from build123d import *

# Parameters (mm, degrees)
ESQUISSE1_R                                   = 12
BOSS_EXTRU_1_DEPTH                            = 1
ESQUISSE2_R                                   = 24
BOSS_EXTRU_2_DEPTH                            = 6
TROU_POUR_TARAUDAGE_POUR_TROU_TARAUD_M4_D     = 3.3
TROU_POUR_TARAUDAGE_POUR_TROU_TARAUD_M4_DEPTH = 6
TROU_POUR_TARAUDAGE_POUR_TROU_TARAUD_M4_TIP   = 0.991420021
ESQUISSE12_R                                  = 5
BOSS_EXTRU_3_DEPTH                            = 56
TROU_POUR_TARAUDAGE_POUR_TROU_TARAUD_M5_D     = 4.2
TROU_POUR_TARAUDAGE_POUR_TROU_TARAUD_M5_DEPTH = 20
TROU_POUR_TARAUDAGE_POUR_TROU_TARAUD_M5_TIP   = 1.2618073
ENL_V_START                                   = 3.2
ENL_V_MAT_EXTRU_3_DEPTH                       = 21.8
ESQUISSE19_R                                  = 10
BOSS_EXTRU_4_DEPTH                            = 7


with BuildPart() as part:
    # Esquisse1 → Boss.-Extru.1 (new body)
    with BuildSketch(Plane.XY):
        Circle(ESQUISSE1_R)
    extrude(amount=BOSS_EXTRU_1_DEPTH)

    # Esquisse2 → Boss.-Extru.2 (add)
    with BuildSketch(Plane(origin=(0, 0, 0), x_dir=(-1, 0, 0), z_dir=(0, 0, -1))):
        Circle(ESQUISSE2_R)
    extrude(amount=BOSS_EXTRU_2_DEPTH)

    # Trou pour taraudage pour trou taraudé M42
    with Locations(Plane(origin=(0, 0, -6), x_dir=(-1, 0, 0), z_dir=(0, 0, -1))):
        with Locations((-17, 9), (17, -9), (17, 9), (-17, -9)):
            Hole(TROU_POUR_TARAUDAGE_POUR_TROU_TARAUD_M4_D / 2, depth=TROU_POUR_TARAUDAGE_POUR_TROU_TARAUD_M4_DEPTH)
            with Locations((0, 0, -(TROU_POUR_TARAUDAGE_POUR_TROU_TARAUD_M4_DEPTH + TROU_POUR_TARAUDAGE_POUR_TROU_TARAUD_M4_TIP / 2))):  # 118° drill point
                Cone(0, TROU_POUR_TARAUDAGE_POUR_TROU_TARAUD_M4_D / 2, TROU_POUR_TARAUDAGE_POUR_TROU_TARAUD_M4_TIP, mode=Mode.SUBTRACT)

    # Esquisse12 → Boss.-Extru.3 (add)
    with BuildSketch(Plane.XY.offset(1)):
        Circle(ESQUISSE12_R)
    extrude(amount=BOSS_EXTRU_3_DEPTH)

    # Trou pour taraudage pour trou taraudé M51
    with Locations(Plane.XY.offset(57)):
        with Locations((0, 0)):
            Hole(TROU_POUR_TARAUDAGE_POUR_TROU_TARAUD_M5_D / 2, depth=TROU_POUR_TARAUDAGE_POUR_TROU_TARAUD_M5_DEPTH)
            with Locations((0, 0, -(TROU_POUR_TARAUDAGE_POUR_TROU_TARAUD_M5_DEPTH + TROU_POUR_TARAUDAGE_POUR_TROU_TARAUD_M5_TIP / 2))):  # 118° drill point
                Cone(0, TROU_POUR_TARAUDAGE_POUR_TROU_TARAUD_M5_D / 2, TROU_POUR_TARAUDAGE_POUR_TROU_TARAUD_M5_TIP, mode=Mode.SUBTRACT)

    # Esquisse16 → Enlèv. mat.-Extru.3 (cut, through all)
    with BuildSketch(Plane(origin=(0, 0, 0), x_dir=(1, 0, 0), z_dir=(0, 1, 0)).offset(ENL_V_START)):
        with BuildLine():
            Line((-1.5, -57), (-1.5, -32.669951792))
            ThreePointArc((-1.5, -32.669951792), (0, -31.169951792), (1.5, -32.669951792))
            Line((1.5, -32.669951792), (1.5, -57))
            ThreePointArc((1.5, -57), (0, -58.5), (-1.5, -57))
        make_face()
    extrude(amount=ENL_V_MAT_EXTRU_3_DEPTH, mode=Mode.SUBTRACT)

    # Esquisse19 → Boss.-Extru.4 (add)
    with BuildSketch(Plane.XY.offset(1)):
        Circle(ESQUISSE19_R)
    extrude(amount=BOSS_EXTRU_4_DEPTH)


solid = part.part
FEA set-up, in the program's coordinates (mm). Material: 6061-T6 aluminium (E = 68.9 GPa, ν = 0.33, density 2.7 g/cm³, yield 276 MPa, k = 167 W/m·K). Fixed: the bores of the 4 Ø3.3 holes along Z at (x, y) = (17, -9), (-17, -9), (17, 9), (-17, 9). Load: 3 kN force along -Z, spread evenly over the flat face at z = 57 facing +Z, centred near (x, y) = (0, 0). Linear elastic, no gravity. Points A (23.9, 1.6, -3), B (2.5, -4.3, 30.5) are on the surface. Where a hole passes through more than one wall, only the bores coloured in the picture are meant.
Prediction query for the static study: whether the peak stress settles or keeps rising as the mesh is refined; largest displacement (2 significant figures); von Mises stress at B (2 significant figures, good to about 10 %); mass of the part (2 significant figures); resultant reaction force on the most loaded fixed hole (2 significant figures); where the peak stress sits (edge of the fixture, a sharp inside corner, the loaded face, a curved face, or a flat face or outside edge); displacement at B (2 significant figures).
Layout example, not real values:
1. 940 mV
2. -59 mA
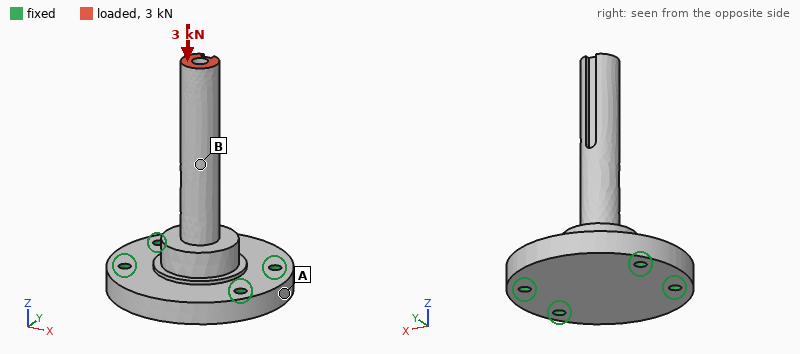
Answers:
1. keeps rising
2. 58 µm
3. 46 MPa
4. 45 g
5. 820 N
6. edge of the fixture
7. 30 µm
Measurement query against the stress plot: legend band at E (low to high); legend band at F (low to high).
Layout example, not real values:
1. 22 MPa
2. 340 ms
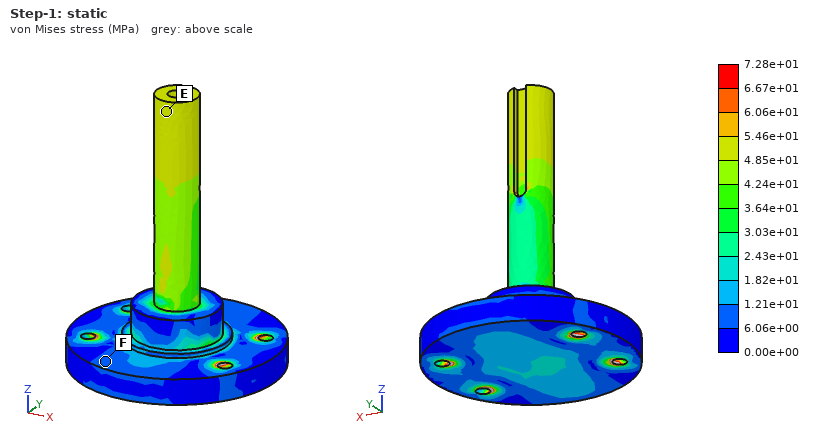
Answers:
1. 4.85e+01 to 5.46e+01 MPa
2. 6.06e+00 to 1.21e+01 MPa
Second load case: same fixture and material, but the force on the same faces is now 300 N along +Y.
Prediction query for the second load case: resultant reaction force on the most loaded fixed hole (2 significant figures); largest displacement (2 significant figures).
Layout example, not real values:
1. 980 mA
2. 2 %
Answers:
1. 430 N
2. 0.46 mm
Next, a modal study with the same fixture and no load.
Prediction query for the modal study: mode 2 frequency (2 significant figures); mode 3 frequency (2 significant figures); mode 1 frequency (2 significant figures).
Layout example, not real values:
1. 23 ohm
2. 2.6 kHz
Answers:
1. 2900 Hz
2. 12 kHz
3. 2800 Hz
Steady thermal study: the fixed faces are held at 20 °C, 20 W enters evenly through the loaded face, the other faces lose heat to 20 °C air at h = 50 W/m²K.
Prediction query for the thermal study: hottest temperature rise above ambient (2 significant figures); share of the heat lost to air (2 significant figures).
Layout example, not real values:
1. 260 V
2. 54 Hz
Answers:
1. 81 K
2. 23 %
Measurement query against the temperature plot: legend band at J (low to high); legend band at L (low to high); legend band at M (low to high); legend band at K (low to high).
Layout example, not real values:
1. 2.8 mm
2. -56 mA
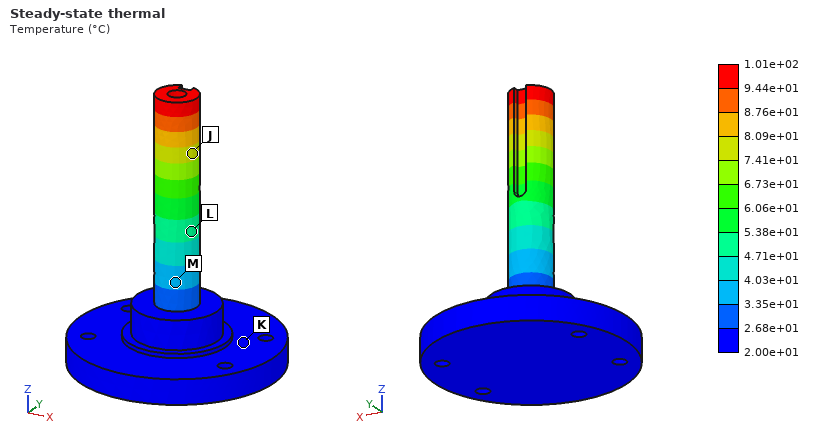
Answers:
1. 7.41e+01 to 8.09e+01 °C
2. 4.71e+01 to 5.38e+01 °C
3. 3.35e+01 to 4.03e+01 °C
4. 2.00e+01 to 2.68e+01 °C
